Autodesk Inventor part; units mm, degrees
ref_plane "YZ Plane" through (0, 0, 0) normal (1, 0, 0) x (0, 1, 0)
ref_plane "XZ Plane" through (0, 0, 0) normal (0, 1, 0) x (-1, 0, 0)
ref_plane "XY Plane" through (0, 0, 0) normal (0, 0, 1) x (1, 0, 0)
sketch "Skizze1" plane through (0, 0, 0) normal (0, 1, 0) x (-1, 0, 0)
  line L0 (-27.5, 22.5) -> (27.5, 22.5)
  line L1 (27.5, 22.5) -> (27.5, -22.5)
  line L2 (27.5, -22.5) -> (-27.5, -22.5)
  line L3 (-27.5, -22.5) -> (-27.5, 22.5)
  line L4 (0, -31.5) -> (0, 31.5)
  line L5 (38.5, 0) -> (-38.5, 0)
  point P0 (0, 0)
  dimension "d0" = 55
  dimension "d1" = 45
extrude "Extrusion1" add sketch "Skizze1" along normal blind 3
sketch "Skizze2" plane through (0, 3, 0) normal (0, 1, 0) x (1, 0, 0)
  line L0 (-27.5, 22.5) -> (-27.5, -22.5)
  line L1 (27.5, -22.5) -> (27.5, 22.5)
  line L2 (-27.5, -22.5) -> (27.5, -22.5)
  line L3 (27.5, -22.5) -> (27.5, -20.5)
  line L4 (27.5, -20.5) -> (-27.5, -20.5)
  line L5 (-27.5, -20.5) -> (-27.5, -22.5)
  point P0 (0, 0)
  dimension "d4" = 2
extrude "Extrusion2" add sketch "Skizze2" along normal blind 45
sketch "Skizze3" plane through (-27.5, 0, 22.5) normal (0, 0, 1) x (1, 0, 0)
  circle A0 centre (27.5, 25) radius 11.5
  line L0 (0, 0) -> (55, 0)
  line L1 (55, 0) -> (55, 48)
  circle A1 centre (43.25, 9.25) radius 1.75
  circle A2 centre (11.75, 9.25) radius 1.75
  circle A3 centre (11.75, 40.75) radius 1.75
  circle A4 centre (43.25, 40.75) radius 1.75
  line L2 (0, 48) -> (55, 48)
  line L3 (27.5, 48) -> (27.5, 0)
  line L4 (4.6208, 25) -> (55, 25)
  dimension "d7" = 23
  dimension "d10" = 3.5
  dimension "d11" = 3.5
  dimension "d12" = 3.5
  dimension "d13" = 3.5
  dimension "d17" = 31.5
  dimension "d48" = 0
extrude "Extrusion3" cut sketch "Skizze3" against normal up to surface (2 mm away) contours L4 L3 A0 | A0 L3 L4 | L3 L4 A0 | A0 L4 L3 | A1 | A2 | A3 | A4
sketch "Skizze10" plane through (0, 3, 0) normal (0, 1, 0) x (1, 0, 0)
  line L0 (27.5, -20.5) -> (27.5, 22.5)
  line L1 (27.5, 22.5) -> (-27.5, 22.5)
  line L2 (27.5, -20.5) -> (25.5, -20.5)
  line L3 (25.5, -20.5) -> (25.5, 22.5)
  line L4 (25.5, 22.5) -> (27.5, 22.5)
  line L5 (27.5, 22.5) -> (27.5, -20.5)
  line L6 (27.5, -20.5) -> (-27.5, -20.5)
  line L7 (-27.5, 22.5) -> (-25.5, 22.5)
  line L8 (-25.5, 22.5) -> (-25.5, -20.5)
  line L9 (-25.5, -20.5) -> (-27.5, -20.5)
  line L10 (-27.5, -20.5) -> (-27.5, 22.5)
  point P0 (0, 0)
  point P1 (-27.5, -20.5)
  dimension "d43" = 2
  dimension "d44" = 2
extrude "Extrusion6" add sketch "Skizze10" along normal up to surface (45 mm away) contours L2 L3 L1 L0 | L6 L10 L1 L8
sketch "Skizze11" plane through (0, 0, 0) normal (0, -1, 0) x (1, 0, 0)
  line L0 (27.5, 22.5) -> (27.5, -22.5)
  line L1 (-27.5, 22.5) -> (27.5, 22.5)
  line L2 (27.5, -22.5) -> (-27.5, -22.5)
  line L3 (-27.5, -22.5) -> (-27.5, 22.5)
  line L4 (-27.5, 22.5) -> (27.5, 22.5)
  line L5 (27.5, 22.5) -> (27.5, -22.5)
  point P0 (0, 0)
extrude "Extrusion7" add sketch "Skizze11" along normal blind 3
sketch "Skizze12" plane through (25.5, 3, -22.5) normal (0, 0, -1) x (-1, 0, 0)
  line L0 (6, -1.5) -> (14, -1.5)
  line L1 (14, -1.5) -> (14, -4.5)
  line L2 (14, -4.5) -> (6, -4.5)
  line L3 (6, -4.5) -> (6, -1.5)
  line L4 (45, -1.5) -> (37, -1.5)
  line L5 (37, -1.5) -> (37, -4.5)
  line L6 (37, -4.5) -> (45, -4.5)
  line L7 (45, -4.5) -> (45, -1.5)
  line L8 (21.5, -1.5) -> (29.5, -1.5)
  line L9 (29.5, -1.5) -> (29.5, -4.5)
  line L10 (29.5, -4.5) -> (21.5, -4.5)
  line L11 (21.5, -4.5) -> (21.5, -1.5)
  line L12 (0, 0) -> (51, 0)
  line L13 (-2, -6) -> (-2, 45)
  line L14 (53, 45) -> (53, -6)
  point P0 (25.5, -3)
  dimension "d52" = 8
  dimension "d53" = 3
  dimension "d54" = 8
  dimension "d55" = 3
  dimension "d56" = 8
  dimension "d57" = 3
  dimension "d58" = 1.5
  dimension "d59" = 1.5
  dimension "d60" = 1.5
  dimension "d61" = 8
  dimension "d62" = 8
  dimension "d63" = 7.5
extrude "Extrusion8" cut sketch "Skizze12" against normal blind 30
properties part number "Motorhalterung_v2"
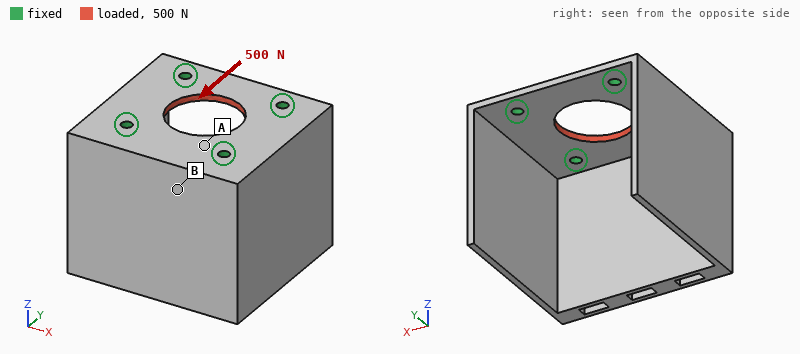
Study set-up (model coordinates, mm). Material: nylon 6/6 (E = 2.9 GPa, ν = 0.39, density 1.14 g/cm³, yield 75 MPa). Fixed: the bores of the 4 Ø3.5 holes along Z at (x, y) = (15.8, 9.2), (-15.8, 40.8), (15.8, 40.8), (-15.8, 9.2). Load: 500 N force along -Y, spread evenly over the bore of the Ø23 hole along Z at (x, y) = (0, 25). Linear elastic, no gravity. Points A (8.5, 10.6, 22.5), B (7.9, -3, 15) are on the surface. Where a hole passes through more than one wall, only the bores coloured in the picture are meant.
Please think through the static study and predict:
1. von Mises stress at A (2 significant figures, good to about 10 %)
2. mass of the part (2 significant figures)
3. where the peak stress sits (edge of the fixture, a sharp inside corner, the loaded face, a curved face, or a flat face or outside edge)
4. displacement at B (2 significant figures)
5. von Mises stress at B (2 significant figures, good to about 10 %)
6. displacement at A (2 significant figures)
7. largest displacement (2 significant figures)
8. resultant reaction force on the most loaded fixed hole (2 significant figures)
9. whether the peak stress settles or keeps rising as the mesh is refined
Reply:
2.9 MPa
28 g
edge of the fixture
13 µm
0.82 MPa
18 µm
49 µm
130 N
keeps rising
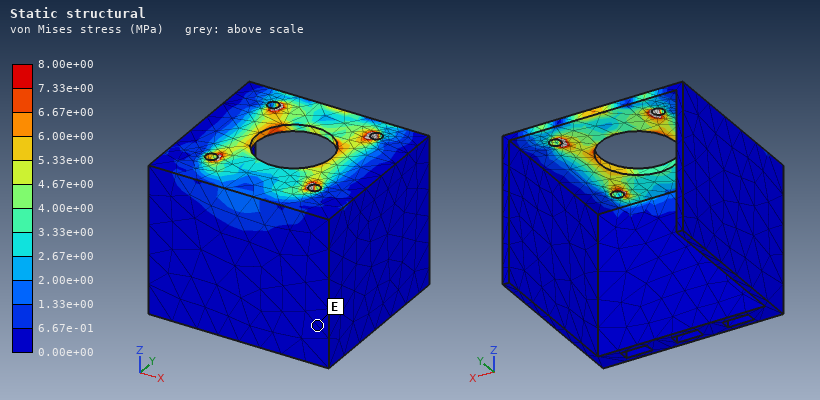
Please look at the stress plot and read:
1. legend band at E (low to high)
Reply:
0.00e+00 to 6.67e-01 MPa
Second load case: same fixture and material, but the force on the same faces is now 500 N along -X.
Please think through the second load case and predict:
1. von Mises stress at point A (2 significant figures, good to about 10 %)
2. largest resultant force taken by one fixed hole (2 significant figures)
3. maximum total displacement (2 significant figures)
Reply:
4.2 MPa
130 N
35 µm
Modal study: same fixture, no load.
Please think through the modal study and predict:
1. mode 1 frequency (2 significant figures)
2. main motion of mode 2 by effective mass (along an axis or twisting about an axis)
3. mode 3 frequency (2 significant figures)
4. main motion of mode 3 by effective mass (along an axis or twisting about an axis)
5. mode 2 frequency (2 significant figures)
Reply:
430 Hz
along X
690 Hz
along Y
450 Hz
